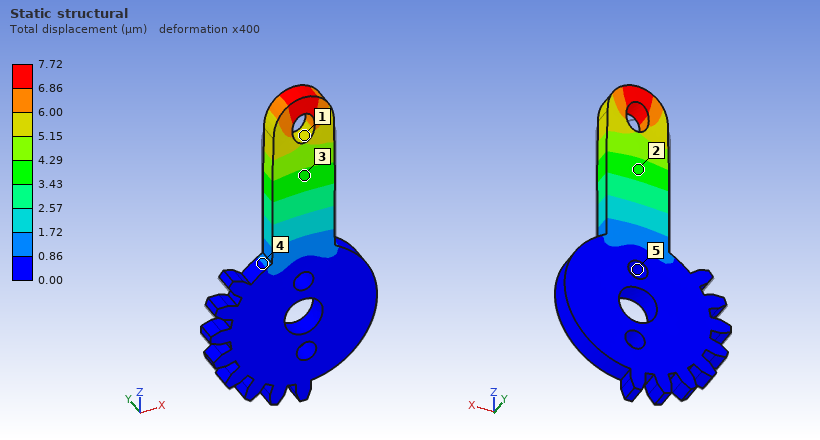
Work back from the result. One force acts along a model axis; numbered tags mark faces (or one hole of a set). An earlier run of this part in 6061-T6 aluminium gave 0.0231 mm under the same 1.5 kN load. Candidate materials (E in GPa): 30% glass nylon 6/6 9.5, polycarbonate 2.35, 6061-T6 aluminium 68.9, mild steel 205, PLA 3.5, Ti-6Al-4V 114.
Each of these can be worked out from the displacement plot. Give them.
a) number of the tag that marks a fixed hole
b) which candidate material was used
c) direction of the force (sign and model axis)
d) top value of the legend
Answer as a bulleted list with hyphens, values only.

- 5
- mild steel
- +Z
- 7.72 µm
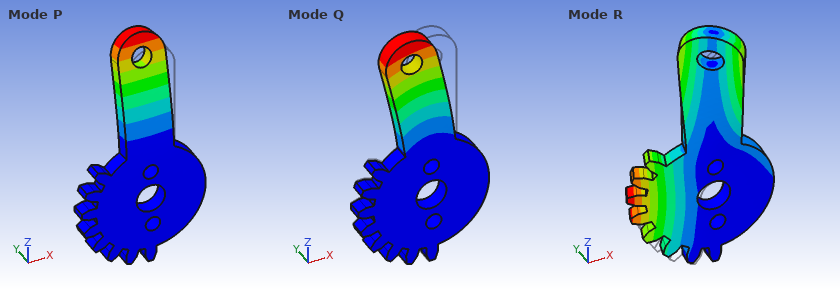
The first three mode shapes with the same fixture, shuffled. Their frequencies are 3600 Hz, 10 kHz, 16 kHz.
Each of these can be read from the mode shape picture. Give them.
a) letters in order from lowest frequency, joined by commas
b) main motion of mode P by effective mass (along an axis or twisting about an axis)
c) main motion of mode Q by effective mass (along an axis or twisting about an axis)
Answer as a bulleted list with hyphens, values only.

- P, Q, R
- along Y
- along X
